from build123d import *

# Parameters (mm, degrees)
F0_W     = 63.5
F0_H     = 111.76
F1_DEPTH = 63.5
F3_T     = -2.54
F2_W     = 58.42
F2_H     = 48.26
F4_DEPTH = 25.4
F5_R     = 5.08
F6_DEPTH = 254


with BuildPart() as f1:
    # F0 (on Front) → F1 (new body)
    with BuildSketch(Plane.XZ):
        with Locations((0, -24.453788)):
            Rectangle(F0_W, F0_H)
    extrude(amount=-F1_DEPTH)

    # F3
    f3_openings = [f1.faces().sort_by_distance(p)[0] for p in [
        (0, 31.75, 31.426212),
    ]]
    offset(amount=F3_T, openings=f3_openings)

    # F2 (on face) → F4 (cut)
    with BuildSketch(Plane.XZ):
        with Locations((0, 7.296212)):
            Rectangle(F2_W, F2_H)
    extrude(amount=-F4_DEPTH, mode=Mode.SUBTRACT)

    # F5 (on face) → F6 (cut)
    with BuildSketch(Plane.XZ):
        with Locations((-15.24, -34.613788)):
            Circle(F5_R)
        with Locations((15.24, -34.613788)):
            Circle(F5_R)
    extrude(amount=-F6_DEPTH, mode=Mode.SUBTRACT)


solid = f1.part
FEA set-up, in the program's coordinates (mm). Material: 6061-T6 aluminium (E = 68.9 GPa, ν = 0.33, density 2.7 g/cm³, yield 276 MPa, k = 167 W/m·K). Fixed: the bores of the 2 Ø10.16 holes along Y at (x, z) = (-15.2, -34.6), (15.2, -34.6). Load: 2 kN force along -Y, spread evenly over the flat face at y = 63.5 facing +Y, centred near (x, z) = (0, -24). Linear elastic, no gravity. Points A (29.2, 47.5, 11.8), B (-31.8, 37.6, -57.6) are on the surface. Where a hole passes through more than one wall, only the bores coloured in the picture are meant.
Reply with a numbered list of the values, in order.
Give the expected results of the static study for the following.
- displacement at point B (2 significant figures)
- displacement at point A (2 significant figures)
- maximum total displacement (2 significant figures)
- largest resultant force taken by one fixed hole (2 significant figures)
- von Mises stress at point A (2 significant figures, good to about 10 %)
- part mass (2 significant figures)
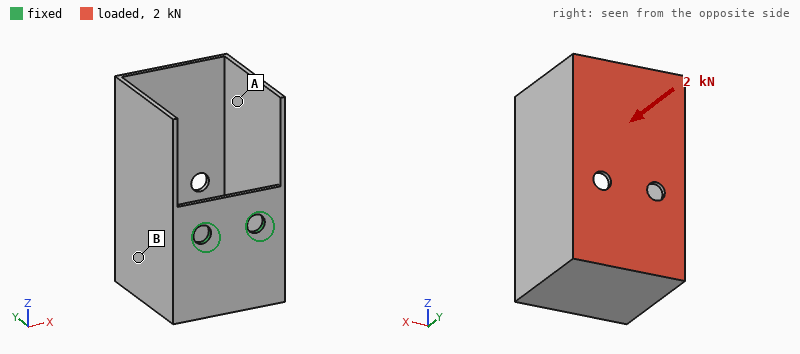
1. 0.47 mm
2. 0.94 mm
3. 1.5 mm
4. 1.0 kN
5. 37 MPa
6. 190 g
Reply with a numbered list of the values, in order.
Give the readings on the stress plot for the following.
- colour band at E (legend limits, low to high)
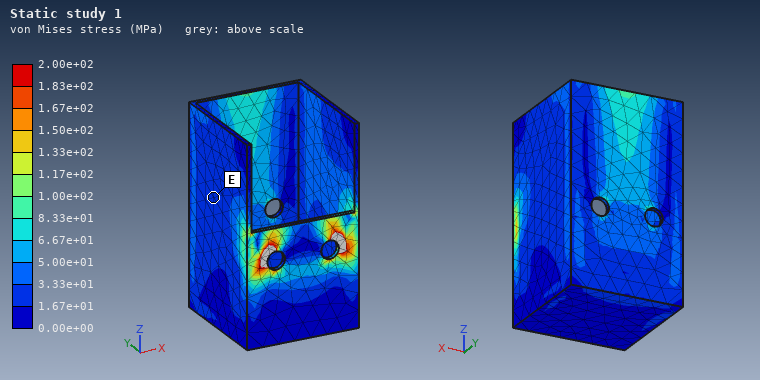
1. 1.67e+01 to 3.33e+01 MPa
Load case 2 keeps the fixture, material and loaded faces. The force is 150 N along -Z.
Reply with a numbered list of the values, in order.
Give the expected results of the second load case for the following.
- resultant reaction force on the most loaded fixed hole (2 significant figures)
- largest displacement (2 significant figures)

1. 76 N
2. 0.44 mm
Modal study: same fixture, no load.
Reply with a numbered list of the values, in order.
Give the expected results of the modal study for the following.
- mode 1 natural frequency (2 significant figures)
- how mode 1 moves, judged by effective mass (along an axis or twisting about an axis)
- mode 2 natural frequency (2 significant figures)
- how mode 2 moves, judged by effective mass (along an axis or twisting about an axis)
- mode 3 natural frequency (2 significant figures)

1. 300 Hz
2. along Z
3. 330 Hz
4. along X
5. 1000 Hz
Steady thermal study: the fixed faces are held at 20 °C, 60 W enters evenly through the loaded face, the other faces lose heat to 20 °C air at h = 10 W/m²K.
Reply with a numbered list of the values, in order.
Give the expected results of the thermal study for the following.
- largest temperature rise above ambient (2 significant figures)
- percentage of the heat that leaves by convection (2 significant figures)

1. 63 K
2. 29 %
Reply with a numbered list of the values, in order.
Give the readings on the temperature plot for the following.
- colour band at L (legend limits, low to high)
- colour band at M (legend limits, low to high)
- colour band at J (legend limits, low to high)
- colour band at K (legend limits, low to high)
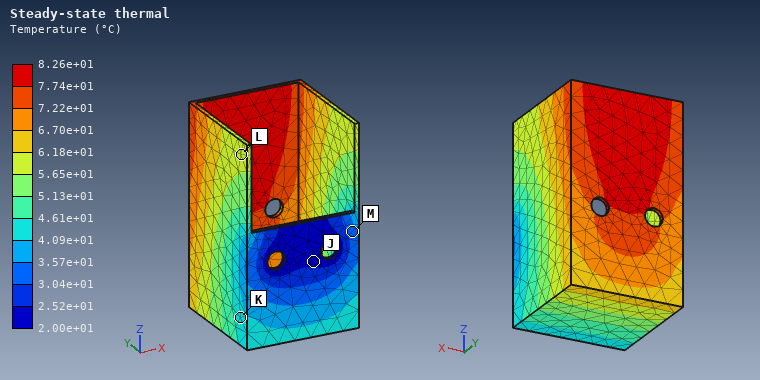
1. 5.65e+01 to 6.18e+01 °C
2. 3.04e+01 to 3.57e+01 °C
3. 2.00e+01 to 2.52e+01 °C
4. 4.09e+01 to 4.61e+01 °C
